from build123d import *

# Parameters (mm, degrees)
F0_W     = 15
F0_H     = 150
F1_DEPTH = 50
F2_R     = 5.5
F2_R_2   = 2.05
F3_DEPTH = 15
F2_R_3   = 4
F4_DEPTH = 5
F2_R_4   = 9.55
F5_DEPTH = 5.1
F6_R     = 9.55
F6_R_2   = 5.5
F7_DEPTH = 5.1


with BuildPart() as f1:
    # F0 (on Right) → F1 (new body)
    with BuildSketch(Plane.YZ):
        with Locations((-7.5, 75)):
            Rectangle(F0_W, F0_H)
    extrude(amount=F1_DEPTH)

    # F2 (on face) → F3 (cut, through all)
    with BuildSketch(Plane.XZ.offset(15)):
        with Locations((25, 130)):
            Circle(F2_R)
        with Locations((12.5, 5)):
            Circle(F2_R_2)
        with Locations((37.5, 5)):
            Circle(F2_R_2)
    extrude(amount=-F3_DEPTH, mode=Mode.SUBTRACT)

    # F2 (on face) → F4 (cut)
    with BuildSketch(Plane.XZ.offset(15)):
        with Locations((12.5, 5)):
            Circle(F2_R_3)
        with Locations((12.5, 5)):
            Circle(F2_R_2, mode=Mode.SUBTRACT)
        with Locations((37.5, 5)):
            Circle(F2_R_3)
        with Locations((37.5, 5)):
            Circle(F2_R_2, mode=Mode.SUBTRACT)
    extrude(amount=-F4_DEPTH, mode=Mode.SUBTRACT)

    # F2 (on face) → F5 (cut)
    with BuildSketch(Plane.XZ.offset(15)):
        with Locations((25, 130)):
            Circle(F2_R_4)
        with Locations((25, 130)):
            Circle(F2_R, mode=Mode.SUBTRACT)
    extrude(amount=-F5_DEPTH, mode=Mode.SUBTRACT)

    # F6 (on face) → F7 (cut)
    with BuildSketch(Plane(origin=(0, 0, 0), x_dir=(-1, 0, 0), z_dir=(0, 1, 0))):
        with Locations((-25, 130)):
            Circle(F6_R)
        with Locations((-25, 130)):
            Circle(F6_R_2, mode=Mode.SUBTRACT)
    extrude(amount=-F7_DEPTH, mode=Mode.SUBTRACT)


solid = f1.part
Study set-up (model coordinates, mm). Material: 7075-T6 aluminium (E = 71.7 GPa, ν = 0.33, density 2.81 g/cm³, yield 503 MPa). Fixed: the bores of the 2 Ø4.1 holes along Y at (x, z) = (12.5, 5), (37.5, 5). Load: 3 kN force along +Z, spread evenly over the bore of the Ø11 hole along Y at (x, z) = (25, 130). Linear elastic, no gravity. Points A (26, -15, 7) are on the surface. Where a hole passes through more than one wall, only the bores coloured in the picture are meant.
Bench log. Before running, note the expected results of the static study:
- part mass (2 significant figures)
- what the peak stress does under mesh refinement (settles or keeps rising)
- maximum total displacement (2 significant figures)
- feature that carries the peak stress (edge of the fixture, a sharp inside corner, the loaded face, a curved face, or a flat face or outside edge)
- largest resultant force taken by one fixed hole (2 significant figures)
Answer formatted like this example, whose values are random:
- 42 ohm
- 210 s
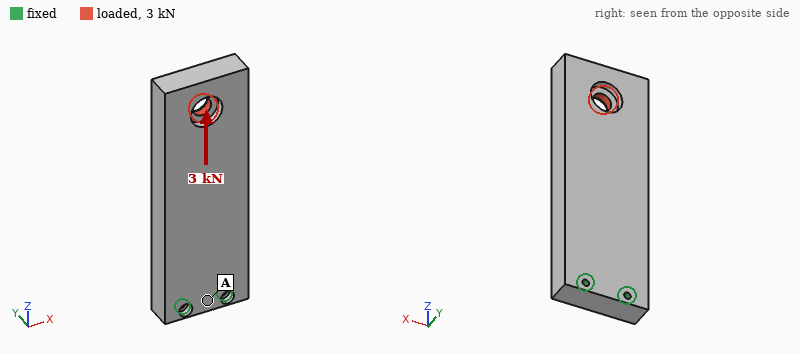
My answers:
- 300 g
- keeps rising
- 28 µm
- edge of the fixture
- 1.5 kN
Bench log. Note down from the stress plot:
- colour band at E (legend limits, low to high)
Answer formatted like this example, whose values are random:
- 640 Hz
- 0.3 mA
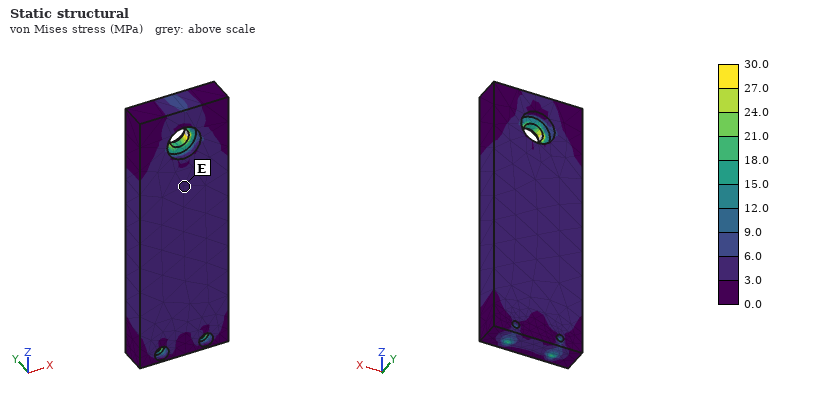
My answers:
- 3.0 to 6.0 MPa
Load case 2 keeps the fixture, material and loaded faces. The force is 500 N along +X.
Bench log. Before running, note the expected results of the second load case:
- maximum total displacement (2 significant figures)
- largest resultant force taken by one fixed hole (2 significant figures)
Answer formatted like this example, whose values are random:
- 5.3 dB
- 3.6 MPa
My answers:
- 63 µm
- 2.3 kN
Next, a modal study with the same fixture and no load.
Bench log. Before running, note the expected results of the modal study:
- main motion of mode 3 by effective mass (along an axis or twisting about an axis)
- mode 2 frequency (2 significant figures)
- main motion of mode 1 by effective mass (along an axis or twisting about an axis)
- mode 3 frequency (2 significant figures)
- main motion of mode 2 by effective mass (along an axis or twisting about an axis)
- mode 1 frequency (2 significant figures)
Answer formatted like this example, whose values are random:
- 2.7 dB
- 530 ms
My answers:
- twisting about Z
- 1400 Hz
- along Y
- 2800 Hz
- along X
- 480 Hz
